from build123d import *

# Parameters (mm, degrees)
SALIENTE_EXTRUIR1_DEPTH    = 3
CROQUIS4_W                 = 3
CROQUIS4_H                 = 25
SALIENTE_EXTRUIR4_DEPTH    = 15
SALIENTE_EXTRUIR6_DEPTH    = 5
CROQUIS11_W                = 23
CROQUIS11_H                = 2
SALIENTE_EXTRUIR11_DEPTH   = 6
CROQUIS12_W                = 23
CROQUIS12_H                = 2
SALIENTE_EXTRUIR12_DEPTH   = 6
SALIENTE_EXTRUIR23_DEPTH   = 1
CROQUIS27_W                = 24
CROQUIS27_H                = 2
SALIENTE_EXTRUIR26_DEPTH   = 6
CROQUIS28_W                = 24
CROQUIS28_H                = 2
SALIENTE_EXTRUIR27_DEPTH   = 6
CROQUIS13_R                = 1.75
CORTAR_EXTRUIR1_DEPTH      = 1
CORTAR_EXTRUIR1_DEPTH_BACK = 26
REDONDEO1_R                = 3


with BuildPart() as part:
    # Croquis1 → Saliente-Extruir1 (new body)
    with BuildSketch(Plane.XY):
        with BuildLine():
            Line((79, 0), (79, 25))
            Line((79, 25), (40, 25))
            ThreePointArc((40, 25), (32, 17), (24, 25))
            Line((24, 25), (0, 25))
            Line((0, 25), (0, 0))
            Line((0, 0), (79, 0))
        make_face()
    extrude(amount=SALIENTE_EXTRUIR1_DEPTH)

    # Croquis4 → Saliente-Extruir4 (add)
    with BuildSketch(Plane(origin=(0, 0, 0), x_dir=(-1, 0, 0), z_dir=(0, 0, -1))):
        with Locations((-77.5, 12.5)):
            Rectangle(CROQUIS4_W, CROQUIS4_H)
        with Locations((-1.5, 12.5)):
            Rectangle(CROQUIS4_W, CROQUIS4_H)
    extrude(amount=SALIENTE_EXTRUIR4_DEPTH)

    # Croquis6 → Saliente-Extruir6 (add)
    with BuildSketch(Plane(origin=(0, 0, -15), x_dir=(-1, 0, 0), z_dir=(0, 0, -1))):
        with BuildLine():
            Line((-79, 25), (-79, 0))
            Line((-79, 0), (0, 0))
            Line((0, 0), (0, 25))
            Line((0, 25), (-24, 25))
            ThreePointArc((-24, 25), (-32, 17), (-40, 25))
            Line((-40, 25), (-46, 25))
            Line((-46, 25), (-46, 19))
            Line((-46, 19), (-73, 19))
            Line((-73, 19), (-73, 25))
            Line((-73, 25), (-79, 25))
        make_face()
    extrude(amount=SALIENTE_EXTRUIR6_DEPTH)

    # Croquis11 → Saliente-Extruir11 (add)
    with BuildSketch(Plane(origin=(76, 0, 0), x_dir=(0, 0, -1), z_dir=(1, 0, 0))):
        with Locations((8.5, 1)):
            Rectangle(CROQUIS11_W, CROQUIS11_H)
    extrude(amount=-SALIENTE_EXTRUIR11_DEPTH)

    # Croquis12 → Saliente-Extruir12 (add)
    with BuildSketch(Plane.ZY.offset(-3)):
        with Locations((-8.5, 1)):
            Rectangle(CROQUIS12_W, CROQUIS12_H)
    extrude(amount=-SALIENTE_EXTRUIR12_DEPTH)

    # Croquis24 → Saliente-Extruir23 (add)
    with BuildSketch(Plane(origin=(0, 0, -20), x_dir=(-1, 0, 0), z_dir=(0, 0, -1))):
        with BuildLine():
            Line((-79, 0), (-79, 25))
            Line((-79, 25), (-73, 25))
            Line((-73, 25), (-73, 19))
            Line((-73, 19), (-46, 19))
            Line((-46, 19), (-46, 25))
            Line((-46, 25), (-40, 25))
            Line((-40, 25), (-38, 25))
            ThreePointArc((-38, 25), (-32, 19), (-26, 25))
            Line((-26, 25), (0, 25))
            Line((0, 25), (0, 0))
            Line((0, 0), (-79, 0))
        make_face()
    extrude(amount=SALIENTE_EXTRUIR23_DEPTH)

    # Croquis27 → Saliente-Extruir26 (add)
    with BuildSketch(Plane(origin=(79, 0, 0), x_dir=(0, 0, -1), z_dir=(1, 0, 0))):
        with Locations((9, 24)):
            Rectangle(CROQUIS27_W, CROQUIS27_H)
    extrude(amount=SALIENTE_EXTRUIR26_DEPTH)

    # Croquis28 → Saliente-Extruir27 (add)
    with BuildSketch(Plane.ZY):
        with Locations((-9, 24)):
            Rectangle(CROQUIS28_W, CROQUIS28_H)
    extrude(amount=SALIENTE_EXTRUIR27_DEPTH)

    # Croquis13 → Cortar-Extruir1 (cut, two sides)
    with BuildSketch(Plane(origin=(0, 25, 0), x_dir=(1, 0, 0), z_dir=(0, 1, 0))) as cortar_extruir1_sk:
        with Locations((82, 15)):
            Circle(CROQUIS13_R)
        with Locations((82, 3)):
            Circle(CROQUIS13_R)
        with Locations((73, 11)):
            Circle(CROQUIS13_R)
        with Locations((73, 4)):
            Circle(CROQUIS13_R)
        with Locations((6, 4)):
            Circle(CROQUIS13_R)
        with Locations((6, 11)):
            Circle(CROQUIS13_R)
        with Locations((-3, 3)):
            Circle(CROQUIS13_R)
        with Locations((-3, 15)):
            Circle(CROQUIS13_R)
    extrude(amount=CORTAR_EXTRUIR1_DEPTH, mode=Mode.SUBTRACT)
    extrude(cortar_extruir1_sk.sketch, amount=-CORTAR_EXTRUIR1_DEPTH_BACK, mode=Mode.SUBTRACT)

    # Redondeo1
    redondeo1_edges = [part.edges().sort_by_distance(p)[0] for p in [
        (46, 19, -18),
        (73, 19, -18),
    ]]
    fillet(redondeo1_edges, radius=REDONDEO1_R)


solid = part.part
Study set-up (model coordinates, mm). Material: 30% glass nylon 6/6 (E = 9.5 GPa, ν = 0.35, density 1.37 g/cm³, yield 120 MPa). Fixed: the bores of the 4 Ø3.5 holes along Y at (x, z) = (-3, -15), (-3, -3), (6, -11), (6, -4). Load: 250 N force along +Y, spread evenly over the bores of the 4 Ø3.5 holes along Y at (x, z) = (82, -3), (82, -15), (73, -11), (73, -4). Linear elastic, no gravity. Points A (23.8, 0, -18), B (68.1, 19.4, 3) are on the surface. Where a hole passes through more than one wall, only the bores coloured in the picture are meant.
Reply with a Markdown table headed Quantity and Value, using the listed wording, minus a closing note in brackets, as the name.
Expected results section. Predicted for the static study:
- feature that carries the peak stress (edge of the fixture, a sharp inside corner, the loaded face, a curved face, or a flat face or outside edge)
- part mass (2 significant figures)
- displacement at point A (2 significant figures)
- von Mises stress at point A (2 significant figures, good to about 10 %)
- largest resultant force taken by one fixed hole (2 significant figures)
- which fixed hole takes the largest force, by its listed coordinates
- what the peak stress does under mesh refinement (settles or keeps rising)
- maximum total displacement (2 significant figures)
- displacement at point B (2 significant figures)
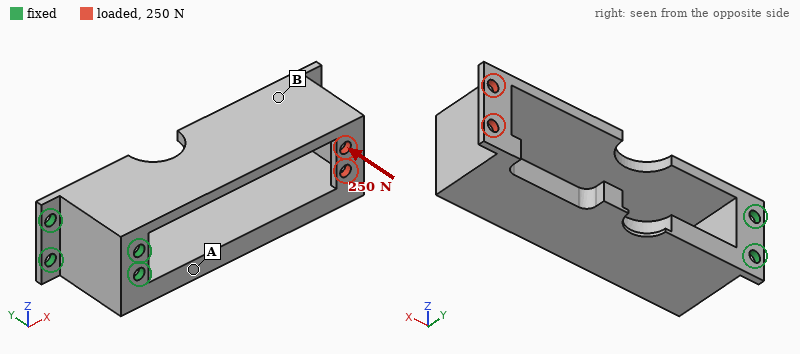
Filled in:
| Quantity | Value |
|---|---|
| feature that carries the peak stress | edge of the fixture |
| part mass | 26 g |
| displacement at point A | 0.18 mm |
| von Mises stress at point A | 20 MPa |
| largest resultant force taken by one fixed hole | 550 N |
| which fixed hole takes the largest force, by its listed coordinates | (6, -11) |
| what the peak stress does under mesh refinement | keeps rising |
| maximum total displacement | 1.0 mm |
| displacement at point B | 0.72 mm |
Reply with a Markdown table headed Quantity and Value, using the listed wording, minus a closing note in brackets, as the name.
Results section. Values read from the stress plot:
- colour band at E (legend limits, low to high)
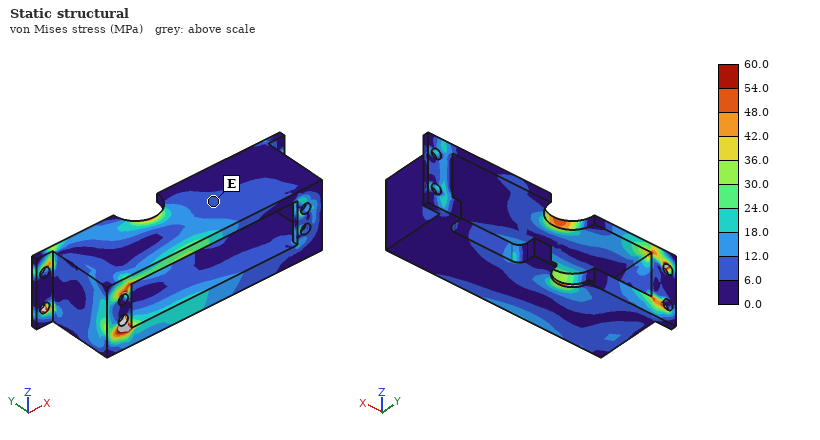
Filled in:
| Quantity | Value |
|---|---|
| colour band at E | 6.0 to 12.0 MPa |
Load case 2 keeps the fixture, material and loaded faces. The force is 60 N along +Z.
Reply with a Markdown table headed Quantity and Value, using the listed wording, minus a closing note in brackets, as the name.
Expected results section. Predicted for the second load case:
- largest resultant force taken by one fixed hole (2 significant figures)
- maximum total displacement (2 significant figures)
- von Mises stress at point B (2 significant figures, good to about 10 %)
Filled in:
| Quantity | Value |
|---|---|
| largest resultant force taken by one fixed hole | 190 N |
| maximum total displacement | 1.0 mm |
| von Mises stress at point B | 7.1 MPa |
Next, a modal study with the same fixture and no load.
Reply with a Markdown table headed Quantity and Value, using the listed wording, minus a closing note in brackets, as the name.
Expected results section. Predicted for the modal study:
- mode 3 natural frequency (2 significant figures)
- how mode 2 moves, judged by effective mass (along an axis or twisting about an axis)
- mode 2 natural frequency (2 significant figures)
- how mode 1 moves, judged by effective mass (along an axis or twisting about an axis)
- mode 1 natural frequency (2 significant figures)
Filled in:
| Quantity | Value |
|---|---|
| mode 3 natural frequency | 1500 Hz |
| how mode 2 moves, judged by effective mass | along Y |
| mode 2 natural frequency | 1000 Hz |
| how mode 1 moves, judged by effective mass | along Z |
| mode 1 natural frequency | 400 Hz |
